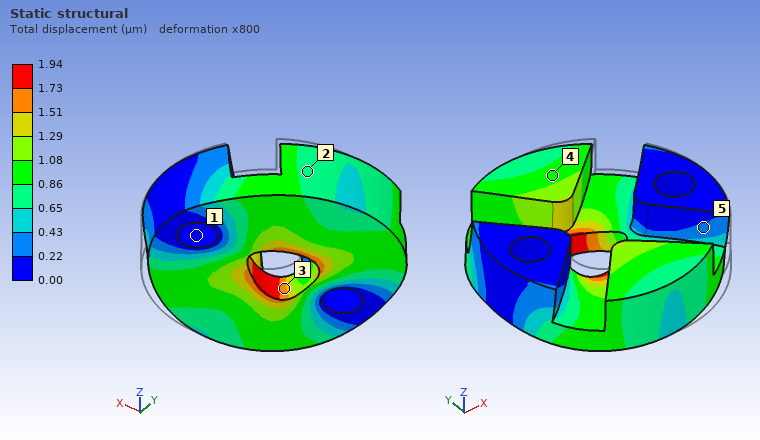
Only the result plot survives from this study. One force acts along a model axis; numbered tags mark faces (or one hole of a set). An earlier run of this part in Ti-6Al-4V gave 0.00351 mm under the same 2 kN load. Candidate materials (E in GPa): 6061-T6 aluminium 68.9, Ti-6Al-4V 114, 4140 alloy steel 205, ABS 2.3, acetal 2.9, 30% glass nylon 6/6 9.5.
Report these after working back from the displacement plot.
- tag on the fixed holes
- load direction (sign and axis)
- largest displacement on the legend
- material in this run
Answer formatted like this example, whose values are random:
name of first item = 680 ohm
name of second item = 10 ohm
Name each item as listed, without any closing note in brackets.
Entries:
tag on the fixed holes = 1
load direction = -X
largest displacement on the legend = 1.94 µm
material in this run = 4140 alloy steel
